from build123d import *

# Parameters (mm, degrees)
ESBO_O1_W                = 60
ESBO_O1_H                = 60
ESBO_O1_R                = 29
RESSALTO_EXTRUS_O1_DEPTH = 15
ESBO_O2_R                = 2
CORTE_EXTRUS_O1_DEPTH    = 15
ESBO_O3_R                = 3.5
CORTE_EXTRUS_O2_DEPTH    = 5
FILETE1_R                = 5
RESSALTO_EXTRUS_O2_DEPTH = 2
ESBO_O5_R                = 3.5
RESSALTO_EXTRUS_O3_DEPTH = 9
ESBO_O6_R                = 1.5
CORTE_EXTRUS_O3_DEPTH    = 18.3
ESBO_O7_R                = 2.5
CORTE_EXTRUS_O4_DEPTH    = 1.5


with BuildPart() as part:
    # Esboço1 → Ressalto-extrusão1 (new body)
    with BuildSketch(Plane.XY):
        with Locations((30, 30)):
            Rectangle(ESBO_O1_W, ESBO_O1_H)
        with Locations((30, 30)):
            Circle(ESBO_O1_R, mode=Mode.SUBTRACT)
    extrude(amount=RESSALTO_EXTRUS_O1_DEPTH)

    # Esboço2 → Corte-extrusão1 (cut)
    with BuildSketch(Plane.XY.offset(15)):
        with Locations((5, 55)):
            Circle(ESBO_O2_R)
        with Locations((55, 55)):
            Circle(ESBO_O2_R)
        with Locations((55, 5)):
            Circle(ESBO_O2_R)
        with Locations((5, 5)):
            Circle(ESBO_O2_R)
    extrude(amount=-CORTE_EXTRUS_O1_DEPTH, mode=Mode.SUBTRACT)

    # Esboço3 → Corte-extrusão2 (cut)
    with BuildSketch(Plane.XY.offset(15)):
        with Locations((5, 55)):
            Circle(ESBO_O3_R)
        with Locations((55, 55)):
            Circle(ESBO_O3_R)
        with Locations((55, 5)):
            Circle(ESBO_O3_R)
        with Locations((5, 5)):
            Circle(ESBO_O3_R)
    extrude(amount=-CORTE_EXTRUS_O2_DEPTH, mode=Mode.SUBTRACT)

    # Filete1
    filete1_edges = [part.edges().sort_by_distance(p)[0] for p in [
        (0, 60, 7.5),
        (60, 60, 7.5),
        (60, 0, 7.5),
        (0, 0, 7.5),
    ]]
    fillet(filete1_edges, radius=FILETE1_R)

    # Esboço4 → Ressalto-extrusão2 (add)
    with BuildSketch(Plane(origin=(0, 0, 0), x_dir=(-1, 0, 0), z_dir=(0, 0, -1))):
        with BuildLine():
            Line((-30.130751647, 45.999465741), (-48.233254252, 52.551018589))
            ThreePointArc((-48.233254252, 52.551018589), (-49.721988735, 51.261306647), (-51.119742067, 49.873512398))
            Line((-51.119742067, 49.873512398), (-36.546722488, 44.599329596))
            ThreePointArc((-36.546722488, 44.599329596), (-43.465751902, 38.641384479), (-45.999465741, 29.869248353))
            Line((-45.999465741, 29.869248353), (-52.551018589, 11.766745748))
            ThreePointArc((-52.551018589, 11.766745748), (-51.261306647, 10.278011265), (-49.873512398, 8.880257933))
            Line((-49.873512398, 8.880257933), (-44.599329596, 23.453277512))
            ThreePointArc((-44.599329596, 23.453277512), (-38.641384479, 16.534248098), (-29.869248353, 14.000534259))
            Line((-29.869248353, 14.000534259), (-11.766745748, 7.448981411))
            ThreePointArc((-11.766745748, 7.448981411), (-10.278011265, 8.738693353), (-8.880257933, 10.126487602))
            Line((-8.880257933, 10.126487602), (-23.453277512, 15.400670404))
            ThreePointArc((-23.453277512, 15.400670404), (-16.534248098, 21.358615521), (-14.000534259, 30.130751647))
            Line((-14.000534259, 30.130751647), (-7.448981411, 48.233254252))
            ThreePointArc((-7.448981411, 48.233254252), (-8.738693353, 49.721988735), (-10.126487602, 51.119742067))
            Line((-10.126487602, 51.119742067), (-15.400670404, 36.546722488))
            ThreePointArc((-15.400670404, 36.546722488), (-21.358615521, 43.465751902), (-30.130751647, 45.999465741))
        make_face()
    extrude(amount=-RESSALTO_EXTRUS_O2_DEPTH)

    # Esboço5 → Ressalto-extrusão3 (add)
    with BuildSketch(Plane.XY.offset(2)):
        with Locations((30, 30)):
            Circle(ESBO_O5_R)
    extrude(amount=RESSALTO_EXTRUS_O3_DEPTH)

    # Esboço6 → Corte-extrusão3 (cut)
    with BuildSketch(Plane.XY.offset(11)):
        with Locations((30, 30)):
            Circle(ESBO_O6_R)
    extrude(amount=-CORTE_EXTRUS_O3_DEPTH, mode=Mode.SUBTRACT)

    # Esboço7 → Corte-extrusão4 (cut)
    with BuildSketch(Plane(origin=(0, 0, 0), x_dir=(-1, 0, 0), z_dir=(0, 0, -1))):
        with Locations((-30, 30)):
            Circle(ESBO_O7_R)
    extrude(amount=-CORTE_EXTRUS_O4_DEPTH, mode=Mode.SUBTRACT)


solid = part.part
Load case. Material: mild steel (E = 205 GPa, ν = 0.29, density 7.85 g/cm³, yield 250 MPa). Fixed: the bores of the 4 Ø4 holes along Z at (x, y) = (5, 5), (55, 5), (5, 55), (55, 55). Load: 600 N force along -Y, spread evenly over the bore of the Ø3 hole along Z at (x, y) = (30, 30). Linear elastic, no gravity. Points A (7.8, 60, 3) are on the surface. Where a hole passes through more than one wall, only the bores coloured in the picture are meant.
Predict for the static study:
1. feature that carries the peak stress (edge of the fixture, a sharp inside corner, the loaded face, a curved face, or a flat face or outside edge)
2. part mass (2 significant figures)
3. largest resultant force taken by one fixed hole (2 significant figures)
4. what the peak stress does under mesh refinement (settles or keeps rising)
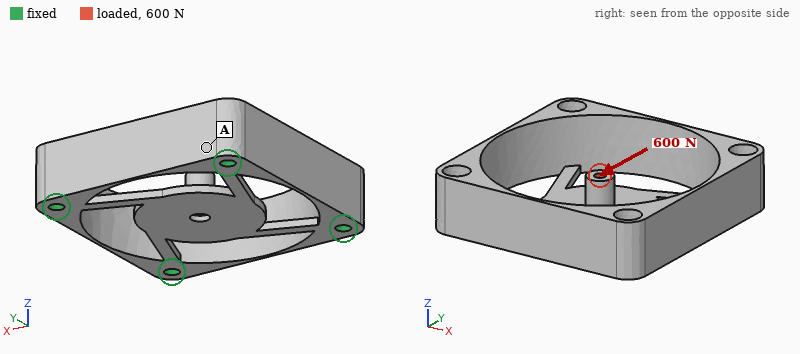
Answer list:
a sharp inside corner
120 g
270 N
keeps rising
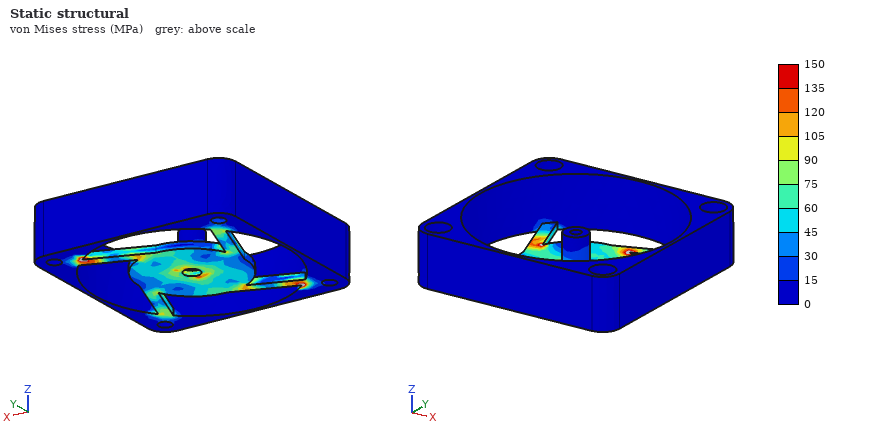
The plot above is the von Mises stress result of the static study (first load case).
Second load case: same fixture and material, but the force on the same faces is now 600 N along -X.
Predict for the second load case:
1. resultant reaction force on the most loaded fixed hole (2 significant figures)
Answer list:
270 N
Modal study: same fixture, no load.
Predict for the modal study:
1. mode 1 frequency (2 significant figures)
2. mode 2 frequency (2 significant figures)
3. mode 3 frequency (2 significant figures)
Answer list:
2200 Hz
4400 Hz
4500 Hz
